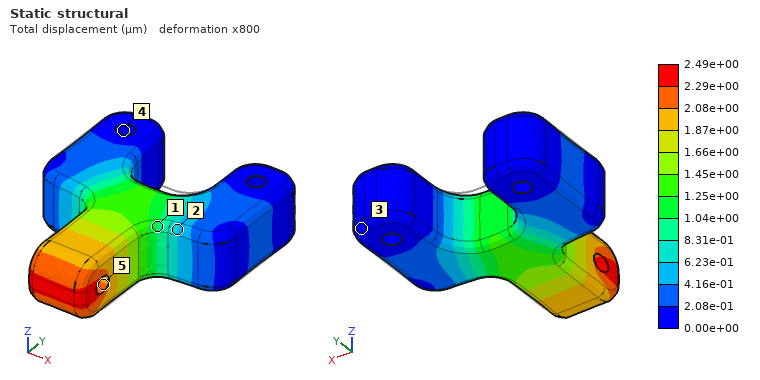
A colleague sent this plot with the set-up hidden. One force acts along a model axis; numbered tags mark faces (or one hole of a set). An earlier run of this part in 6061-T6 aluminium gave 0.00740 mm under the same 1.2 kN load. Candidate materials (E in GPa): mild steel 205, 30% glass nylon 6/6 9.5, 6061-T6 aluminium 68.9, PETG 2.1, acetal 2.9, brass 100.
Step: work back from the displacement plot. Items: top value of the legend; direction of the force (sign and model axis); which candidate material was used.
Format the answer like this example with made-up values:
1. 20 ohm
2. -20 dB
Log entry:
1. 2.49e+00 µm
2. -Y
3. mild steel
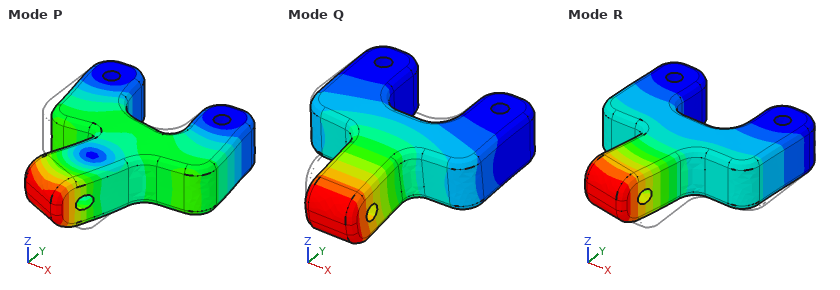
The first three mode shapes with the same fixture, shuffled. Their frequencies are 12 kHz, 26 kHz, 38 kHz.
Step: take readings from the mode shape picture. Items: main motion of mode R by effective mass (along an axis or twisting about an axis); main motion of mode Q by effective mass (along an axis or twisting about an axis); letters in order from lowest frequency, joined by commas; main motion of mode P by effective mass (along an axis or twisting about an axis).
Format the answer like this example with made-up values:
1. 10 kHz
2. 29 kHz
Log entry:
1. along X
2. along Z
3. Q, R, P
4. along X
